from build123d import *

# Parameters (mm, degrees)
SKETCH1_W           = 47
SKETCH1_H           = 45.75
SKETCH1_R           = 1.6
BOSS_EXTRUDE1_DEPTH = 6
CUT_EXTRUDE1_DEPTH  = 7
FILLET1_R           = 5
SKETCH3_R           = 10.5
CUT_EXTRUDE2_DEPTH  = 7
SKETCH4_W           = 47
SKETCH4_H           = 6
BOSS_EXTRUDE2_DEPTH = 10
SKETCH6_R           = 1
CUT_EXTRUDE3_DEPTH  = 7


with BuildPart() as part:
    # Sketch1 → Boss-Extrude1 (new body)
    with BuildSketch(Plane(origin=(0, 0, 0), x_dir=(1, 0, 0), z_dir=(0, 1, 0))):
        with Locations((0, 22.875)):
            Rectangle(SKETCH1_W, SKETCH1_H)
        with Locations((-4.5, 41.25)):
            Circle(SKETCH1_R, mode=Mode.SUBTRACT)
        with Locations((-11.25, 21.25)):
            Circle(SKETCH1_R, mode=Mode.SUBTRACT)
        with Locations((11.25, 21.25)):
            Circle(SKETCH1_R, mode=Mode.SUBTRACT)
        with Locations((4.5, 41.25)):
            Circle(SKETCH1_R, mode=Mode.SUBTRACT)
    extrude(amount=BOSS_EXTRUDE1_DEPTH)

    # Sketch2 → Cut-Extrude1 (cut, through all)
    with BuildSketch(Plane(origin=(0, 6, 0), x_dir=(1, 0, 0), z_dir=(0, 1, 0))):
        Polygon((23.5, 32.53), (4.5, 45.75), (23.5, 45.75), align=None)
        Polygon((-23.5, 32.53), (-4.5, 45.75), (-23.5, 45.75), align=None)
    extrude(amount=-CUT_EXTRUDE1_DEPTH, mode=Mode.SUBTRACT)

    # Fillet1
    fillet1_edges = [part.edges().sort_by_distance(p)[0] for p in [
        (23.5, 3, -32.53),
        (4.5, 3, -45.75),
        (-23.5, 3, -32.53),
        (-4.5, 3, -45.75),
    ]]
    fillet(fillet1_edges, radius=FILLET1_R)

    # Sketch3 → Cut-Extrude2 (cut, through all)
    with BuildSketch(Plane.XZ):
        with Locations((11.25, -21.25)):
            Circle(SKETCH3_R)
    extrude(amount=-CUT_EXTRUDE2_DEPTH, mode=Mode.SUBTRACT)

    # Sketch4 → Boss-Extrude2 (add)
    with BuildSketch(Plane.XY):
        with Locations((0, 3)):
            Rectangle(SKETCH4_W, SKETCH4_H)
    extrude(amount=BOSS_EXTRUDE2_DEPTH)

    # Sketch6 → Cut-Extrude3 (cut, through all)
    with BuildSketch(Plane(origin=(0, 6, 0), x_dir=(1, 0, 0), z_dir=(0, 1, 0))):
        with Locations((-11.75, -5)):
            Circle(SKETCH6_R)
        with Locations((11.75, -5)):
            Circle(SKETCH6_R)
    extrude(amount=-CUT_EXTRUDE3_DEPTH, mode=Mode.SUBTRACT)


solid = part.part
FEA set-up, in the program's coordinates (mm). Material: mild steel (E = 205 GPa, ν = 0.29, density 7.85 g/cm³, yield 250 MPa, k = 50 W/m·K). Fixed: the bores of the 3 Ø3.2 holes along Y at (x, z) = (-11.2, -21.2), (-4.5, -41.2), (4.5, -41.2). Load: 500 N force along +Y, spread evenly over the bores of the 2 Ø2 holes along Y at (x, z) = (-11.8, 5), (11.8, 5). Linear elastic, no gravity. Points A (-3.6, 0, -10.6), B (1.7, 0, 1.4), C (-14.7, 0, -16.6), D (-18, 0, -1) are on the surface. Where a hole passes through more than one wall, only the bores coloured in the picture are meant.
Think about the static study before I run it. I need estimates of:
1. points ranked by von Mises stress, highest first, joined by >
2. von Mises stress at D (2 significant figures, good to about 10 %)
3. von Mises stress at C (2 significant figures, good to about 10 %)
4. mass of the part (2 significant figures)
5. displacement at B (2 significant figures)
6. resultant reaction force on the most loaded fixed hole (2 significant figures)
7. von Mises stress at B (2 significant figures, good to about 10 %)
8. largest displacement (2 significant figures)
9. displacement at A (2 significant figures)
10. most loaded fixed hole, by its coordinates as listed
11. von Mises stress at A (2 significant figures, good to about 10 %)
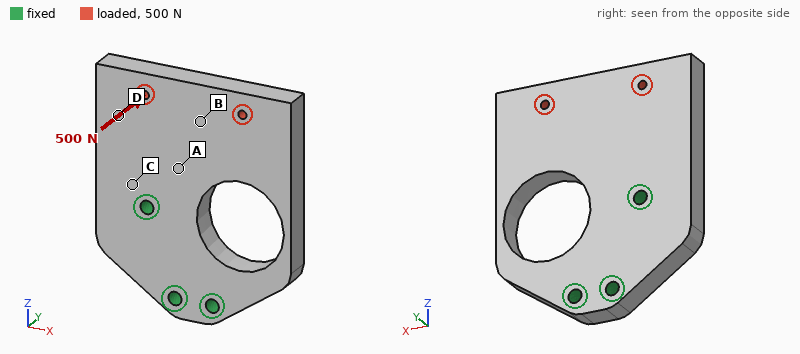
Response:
C > A > D > B
23 MPa
63 MPa
94 g
40 µm
690 N
13 MPa
79 µm
15 µm
(-11.2, -21.2)
43 MPa
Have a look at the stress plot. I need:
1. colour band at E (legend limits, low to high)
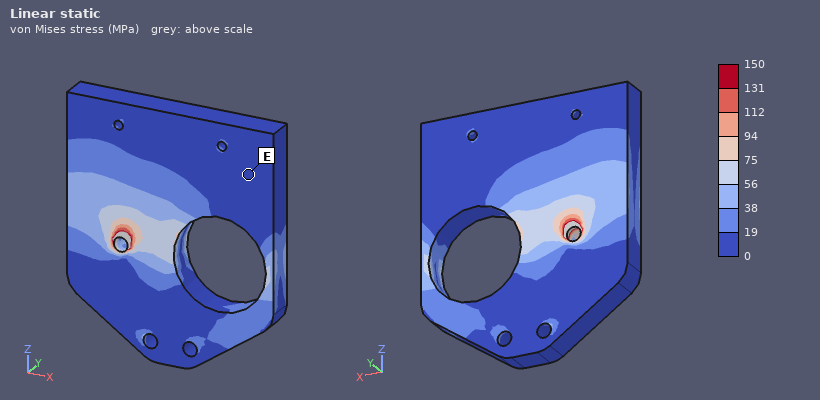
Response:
0 to 19 MPa
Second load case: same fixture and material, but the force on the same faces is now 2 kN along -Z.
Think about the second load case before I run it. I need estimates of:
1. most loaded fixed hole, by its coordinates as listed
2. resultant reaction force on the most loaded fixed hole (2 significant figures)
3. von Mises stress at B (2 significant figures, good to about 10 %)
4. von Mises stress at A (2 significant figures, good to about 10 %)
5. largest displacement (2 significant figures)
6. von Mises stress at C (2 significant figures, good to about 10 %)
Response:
(-11.2, -21.2)
1.2 kN
7.5 MPa
16 MPa
11 µm
11 MPa
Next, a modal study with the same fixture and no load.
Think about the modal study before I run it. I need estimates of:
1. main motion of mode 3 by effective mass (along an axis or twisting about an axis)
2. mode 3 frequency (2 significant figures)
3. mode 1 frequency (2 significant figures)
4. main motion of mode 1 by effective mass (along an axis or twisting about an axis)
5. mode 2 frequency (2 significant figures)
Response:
along X
7500 Hz
2700 Hz
along Y
5500 Hz
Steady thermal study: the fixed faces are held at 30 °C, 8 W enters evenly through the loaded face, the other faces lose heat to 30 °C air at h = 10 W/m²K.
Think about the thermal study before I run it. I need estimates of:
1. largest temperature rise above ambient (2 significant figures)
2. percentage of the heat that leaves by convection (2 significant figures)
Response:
30 K
8.5 %
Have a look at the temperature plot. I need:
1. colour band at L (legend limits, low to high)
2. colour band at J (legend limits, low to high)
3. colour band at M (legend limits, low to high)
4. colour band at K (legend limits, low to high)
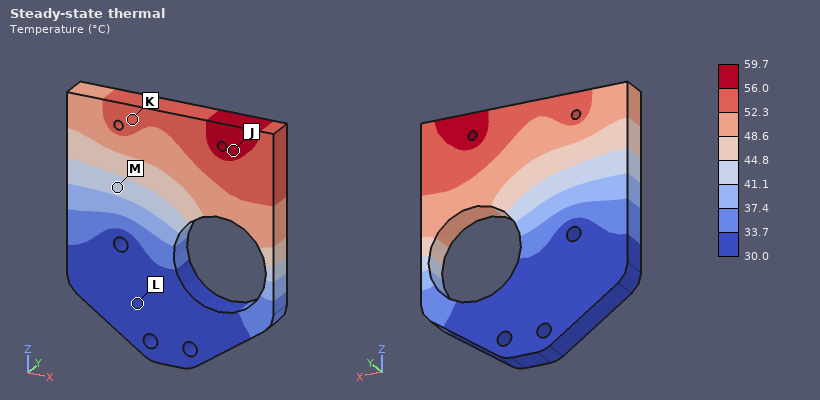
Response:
30.0 to 33.7 °C
56.0 to 59.7 °C
41.1 to 44.8 °C
52.3 to 56.0 °C
